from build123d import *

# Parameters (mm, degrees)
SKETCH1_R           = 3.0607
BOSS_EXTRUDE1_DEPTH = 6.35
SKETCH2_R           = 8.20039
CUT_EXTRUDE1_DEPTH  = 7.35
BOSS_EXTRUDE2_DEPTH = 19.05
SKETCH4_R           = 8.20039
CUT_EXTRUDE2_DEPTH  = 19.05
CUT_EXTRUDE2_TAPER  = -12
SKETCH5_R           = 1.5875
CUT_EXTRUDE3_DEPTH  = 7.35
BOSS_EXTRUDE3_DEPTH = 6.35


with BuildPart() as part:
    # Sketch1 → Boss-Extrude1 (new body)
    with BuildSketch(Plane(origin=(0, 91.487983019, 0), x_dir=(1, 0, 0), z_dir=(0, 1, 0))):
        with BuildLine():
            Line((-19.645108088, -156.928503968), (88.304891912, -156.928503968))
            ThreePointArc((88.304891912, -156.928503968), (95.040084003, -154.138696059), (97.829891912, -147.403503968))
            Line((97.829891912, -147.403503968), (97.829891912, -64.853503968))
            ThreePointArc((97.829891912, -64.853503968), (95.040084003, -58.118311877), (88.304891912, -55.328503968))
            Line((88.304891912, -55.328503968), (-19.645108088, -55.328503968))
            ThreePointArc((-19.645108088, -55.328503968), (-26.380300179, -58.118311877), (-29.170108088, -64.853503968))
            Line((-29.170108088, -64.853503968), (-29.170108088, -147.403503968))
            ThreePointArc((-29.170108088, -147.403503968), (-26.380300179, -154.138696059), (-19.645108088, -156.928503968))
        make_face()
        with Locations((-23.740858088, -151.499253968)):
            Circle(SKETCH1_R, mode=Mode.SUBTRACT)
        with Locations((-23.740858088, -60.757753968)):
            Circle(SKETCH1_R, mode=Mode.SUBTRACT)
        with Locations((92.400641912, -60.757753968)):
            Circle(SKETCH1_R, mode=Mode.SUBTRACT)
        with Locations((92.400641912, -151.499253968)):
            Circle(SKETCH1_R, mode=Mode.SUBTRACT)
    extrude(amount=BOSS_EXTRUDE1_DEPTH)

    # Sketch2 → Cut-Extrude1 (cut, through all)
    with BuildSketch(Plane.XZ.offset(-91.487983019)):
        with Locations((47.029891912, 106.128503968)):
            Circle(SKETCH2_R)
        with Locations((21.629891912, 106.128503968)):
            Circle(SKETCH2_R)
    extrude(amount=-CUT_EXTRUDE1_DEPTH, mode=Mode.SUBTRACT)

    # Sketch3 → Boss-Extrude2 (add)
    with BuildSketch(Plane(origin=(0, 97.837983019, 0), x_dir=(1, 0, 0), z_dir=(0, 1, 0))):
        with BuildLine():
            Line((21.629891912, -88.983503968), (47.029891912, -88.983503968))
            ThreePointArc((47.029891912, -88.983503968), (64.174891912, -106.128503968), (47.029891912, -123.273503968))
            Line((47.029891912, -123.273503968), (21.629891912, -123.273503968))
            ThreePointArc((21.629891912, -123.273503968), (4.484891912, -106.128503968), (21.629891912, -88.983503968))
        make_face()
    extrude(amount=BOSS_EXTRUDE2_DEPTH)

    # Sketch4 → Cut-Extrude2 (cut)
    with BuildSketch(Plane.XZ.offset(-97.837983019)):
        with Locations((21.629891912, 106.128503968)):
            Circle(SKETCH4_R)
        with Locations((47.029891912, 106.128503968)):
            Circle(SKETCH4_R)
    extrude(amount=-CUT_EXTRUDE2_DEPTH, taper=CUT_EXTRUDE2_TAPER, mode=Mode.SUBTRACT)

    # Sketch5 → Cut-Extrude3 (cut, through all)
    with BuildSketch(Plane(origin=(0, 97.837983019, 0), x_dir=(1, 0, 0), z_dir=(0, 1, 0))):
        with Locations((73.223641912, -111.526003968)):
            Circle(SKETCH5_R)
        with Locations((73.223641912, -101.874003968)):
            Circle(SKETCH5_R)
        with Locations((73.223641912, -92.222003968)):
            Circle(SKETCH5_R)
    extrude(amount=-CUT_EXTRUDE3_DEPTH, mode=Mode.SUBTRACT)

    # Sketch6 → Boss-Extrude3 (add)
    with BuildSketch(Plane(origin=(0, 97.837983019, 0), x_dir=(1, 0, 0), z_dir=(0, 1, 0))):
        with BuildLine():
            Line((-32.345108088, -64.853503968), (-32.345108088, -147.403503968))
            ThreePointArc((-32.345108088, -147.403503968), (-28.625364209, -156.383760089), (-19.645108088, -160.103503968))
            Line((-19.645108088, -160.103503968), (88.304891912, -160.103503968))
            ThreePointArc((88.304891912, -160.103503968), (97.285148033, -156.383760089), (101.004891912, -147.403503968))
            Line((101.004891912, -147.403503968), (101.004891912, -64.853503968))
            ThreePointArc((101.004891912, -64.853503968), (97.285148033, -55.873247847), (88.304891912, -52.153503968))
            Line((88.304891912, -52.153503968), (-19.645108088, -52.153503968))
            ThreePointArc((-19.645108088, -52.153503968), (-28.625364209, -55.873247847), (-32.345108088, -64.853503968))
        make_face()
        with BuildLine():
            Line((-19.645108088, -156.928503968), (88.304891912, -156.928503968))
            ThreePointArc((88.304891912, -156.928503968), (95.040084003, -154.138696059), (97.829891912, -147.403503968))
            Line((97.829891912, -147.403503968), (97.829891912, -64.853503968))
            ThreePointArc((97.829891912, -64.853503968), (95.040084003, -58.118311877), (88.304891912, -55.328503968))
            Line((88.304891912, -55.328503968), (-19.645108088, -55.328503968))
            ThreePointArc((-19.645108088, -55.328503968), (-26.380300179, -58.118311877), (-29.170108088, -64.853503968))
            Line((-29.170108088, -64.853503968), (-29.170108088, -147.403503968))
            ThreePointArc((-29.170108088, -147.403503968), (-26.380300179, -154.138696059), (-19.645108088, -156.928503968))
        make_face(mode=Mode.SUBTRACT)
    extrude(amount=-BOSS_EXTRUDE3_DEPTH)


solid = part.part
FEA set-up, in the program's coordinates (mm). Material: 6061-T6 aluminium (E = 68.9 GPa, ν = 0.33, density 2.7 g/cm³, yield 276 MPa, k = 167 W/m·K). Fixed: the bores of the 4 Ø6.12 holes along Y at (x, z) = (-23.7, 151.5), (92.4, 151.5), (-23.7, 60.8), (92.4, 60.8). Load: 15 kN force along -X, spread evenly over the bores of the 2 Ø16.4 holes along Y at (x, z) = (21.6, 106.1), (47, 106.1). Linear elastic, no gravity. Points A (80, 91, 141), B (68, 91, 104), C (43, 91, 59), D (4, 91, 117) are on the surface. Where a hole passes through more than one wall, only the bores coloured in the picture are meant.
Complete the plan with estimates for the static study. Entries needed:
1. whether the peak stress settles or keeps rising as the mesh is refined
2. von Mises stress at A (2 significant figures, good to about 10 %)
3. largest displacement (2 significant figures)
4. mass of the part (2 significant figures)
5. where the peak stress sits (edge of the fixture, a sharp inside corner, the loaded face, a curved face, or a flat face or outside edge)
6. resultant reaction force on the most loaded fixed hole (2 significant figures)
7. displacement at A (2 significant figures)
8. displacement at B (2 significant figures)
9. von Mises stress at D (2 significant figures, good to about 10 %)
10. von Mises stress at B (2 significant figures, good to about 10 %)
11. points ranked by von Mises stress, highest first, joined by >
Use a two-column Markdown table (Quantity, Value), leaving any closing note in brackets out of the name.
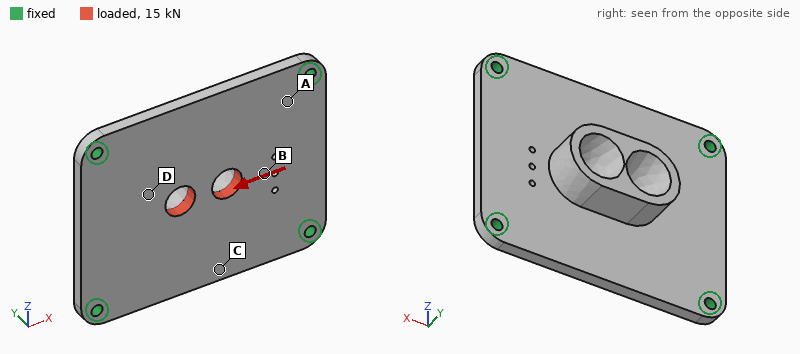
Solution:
| Quantity | Value |
|---|---|
| whether the peak stress settles or keeps rising as the mesh is refined | keeps rising |
| von Mises stress at A | 26 MPa |
| largest displacement | 33 µm |
| mass of the part | 290 g |
| where the peak stress sits | edge of the fixture |
| resultant reaction force on the most loaded fixed hole | 4.1 kN |
| displacement at A | 8.7 µm |
| displacement at B | 20 µm |
| von Mises stress at D | 17 MPa |
| von Mises stress at B | 11 MPa |
| points ranked by von Mises stress, highest first, joined by > | A > D > B > C |
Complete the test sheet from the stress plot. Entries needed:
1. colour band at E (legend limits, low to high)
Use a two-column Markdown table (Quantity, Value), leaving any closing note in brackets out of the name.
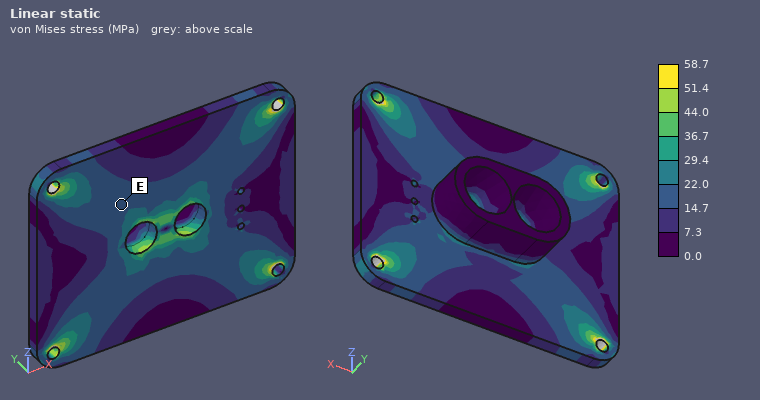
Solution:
| Quantity | Value |
|---|---|
| colour band at E | 14.7 to 22.0 MPa |
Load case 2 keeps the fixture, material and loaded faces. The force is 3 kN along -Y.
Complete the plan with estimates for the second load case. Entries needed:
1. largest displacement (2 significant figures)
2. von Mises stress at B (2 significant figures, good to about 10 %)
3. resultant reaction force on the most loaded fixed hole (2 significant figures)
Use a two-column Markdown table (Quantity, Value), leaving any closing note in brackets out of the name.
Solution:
| Quantity | Value |
|---|---|
| largest displacement | 0.15 mm |
| von Mises stress at B | 40 MPa |
| resultant reaction force on the most loaded fixed hole | 810 N |
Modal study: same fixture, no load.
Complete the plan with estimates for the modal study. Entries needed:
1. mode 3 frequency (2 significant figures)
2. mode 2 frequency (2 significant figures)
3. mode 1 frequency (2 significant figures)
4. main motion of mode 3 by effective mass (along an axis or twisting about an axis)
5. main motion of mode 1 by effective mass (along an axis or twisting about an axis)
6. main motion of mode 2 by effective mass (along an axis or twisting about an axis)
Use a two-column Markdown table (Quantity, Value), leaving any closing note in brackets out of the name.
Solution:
| Quantity | Value |
|---|---|
| mode 3 frequency | 3500 Hz |
| mode 2 frequency | 2800 Hz |
| mode 1 frequency | 1800 Hz |
| main motion of mode 3 by effective mass | twisting about Z |
| main motion of mode 1 by effective mass | along Y |
| main motion of mode 2 by effective mass | twisting about X |
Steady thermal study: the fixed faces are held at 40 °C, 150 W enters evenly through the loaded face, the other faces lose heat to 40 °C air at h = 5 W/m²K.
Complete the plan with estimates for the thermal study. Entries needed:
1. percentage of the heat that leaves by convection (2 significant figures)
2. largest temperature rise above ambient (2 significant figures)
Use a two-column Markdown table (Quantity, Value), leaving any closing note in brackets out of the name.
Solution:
| Quantity | Value |
|---|---|
| percentage of the heat that leaves by convection | 3.5 % |
| largest temperature rise above ambient | 59 K |
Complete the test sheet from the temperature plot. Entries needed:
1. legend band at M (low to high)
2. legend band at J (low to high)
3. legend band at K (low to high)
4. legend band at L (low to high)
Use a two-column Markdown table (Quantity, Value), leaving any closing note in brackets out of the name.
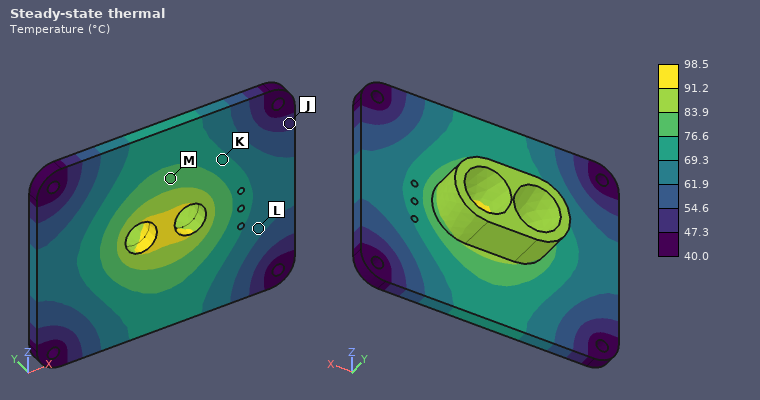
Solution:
| Quantity | Value |
|---|---|
| legend band at M | 76.6 to 83.9 °C |
| legend band at J | 47.3 to 54.6 °C |
| legend band at K | 69.3 to 76.6 °C |
| legend band at L | 61.9 to 69.3 °C |
